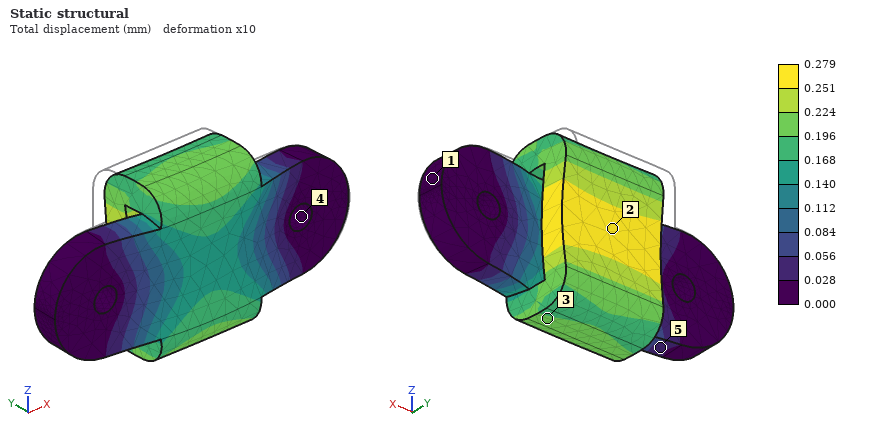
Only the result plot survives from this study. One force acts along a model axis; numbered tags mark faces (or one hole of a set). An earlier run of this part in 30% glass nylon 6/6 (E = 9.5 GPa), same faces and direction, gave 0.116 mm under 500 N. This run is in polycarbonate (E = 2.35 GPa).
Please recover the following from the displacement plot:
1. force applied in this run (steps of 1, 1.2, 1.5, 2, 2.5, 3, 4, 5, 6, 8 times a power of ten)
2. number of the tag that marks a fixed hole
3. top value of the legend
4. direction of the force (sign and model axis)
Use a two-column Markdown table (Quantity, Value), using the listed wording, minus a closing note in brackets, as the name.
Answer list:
| Quantity | Value |
|---|---|
| force applied in this run | 300 N |
| number of the tag that marks a fixed hole | 4 |
| top value of the legend | 0.279 mm |
| direction of the force | -Y |
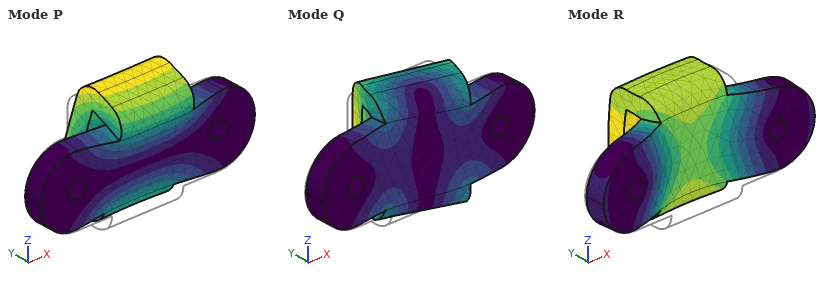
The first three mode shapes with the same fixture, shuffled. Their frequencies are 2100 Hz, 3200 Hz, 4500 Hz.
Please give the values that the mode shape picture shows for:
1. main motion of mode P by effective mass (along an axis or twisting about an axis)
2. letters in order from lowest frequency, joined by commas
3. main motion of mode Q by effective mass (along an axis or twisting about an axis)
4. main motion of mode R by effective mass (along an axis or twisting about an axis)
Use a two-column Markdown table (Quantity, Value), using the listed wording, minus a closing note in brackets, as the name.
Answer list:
| Quantity | Value |
|---|---|
| main motion of mode P by effective mass | along Z |
| letters in order from lowest frequency, joined by commas | P, R, Q |
| main motion of mode Q by effective mass | along X |
| main motion of mode R by effective mass | along Y |
